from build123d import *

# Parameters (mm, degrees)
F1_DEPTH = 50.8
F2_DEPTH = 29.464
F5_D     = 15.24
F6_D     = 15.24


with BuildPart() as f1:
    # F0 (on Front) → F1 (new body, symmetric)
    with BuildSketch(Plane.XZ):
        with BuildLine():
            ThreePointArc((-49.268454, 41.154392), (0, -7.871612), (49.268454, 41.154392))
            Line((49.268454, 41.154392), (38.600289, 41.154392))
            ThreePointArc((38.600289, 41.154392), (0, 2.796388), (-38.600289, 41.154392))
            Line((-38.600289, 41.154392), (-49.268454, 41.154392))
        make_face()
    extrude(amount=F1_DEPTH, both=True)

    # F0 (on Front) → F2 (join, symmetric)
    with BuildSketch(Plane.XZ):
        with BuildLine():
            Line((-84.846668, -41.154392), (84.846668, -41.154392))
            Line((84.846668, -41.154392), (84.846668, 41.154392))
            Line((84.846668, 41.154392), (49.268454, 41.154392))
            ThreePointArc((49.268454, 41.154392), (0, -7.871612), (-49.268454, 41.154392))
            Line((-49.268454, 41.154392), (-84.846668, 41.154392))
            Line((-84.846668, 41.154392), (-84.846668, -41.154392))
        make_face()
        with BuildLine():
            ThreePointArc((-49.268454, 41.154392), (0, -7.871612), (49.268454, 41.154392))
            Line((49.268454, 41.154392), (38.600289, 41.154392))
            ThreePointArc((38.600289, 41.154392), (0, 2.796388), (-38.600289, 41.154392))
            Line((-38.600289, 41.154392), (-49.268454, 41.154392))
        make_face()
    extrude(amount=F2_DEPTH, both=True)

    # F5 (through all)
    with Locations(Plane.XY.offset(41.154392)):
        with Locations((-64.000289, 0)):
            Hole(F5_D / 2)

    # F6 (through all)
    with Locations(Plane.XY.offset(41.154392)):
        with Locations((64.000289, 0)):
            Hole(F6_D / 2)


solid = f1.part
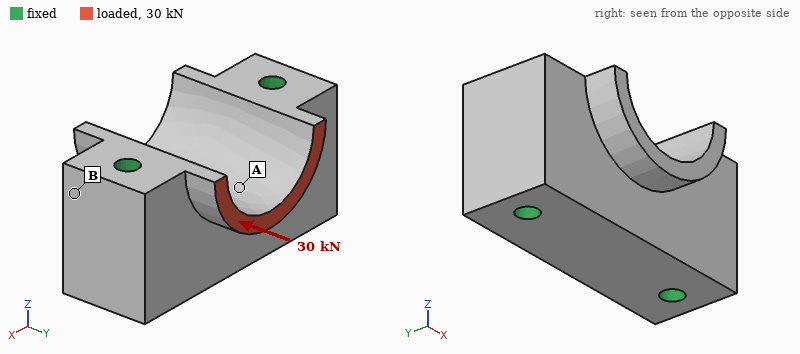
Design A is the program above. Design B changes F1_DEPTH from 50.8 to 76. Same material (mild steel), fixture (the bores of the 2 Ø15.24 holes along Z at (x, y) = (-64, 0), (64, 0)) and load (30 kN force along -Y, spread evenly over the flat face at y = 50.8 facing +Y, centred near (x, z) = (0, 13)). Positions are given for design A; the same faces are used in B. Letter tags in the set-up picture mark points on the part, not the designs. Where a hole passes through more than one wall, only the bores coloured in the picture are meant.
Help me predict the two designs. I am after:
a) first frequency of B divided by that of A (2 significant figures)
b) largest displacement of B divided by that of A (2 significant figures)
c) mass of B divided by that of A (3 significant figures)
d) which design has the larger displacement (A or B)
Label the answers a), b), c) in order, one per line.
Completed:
a) 0.58
b) 1.1
c) 1.10
d) B
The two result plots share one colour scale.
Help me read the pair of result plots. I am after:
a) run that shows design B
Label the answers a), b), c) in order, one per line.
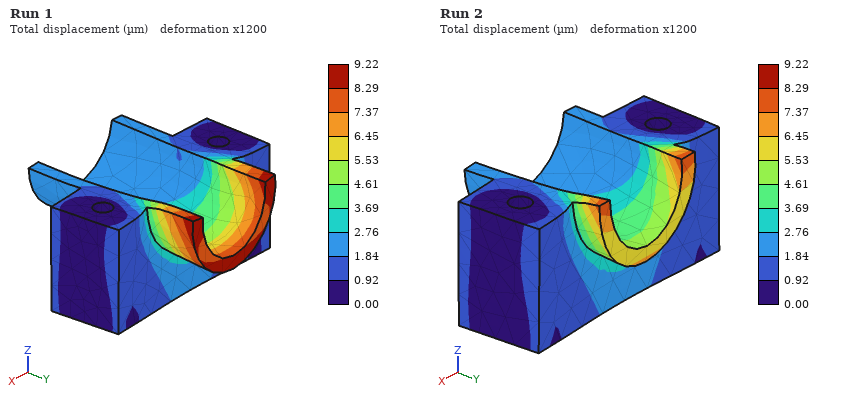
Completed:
a) Run 1
